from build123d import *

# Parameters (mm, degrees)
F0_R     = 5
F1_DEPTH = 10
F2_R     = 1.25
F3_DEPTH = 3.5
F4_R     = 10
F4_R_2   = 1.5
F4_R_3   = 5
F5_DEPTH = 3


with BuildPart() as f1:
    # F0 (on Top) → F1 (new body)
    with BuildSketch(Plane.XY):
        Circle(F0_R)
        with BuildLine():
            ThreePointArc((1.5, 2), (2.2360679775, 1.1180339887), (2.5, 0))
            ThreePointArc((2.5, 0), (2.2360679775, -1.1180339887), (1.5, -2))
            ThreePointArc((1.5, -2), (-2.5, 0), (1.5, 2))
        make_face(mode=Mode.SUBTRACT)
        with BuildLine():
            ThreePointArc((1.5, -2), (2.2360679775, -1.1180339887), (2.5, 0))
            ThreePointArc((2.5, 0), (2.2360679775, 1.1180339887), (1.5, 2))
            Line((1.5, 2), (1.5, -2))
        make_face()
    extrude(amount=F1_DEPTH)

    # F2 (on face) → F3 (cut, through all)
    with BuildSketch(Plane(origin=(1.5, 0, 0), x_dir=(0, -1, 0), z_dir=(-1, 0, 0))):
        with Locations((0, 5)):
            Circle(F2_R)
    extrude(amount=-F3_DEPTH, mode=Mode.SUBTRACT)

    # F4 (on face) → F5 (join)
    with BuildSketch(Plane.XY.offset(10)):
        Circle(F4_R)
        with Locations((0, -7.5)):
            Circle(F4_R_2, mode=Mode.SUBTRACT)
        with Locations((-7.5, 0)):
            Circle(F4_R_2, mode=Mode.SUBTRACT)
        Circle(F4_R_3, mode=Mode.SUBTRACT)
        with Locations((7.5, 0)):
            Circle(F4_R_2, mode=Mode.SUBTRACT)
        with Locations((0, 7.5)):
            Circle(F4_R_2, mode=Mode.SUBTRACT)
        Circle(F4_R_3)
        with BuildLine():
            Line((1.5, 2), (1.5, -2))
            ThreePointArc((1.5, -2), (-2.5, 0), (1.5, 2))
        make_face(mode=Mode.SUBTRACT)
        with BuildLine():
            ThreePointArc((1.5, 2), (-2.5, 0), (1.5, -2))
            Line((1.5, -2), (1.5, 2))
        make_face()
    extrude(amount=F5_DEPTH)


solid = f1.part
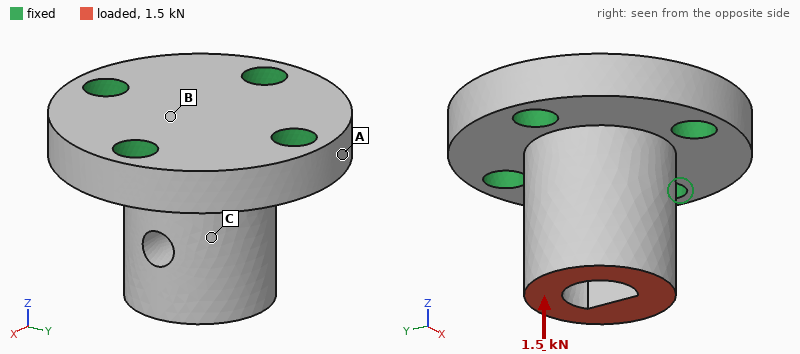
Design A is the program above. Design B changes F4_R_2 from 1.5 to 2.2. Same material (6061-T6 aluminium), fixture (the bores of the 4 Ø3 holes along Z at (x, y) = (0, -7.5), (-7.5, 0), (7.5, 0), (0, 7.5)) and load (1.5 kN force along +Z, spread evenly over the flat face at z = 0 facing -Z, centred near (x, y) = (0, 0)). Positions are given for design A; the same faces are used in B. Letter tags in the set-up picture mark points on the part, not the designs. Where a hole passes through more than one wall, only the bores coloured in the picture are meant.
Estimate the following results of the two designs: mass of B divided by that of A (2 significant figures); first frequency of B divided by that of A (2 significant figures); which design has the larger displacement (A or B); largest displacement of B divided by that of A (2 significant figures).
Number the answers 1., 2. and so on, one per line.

1. 0.93
2. 1.1
3. A
4. 0.85
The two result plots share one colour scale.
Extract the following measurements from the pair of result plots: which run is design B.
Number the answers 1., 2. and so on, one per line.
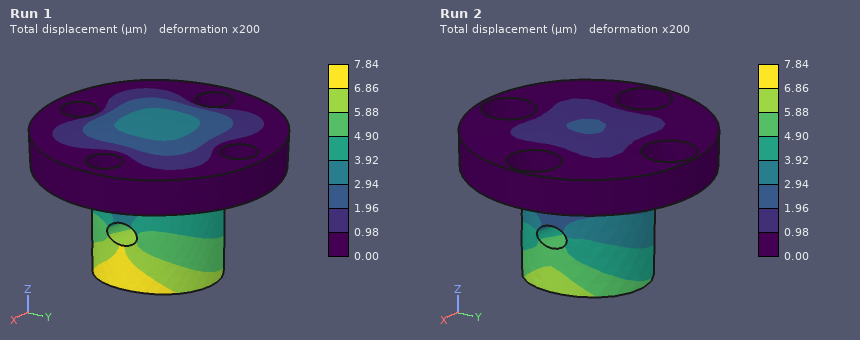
1. Run 2
